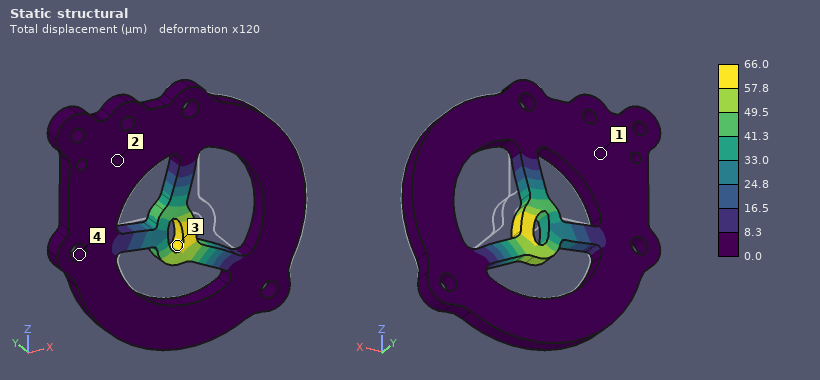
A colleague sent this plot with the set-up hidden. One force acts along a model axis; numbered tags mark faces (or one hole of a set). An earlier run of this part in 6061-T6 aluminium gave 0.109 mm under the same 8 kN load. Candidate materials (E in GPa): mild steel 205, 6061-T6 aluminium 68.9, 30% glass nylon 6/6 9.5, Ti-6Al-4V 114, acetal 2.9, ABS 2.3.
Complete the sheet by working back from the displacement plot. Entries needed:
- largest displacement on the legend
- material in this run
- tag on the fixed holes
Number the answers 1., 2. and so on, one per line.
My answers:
1. 66.0 µm
2. Ti-6Al-4V
3. 4
